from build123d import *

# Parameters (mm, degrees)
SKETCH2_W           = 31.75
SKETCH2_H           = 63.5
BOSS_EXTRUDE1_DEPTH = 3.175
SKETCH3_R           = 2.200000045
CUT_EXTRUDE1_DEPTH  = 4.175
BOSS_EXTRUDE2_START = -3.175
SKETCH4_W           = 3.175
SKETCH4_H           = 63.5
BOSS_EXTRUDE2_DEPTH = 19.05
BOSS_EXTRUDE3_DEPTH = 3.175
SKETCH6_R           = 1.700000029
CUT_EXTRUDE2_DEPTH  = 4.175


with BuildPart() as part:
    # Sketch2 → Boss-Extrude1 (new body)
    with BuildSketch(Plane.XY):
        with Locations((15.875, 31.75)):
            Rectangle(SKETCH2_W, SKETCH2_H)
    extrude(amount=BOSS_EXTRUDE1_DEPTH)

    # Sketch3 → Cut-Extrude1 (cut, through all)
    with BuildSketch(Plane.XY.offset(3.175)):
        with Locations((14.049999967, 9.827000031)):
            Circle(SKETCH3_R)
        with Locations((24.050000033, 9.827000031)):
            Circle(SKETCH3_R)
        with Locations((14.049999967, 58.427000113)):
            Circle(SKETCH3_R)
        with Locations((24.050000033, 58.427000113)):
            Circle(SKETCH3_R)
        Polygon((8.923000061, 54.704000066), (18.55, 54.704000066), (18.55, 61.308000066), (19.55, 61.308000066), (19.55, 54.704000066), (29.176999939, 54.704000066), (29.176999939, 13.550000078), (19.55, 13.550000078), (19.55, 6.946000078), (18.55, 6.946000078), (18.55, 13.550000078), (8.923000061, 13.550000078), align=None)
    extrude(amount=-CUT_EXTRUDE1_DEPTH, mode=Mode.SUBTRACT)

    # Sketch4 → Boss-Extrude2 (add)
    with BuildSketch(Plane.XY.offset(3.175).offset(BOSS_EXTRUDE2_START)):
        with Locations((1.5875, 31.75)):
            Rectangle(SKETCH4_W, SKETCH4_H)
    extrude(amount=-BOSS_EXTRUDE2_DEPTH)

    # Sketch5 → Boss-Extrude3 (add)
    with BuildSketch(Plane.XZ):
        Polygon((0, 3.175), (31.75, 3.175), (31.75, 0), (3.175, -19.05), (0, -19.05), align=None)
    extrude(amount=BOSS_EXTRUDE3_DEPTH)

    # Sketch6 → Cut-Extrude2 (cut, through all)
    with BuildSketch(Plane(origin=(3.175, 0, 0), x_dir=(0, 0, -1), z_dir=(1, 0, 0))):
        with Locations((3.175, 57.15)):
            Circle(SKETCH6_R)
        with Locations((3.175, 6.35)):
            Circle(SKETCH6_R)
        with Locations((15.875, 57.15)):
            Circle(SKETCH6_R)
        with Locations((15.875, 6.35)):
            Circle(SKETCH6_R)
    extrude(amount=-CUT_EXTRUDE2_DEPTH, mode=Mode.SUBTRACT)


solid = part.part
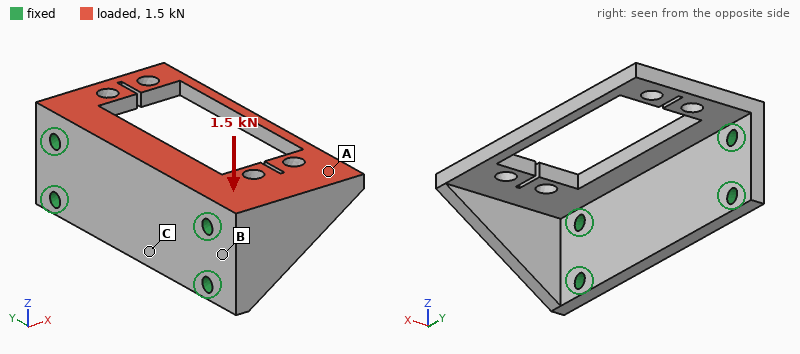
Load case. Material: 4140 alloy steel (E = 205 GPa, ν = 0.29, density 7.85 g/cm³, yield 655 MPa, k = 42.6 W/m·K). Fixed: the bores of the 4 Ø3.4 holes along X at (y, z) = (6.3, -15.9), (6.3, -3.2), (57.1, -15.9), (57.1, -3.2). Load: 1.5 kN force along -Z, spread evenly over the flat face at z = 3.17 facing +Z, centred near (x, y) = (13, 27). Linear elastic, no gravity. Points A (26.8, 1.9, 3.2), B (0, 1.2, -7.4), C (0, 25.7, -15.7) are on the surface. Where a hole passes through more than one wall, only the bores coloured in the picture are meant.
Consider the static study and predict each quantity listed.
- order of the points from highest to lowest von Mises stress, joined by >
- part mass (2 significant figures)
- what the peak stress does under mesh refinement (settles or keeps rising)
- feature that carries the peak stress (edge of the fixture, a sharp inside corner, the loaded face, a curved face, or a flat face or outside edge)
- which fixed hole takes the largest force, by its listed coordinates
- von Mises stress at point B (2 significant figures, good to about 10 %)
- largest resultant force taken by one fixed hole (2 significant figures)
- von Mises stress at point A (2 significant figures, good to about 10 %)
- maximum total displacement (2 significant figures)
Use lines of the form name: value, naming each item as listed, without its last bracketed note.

order of the points from highest to lowest von Mises stress, joined by >: A > B > C
part mass: 68 g
what the peak stress does under mesh refinement: keeps rising
feature that carries the peak stress: a sharp inside corner
which fixed hole takes the largest force, by its listed coordinates: (6.3, -3.2)
von Mises stress at point B: 59 MPa
largest resultant force taken by one fixed hole: 920 N
von Mises stress at point A: 89 MPa
maximum total displacement: 0.37 mm
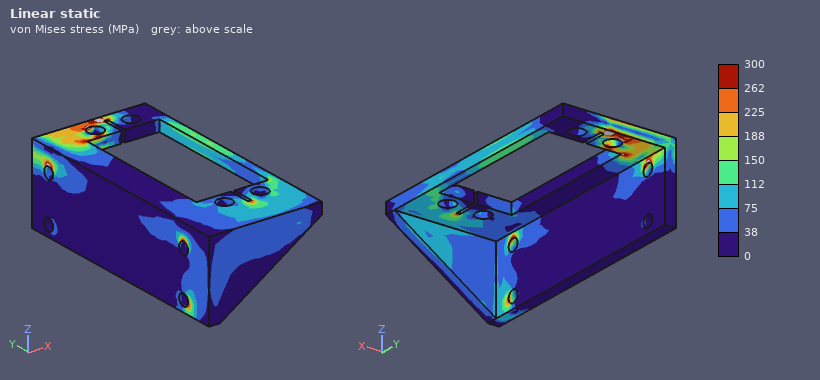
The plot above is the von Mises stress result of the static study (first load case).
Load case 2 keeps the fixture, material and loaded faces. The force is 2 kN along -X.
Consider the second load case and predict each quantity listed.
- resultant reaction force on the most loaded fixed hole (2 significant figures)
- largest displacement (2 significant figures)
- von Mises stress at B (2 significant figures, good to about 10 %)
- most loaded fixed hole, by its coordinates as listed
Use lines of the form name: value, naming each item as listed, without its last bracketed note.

resultant reaction force on the most loaded fixed hole: 1.5 kN
largest displacement: 0.10 mm
von Mises stress at B: 32 MPa
most loaded fixed hole, by its coordinates as listed: (6.3, -3.2)
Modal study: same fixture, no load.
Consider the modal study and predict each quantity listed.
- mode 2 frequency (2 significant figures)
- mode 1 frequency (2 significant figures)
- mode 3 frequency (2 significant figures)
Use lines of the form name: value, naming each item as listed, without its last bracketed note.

mode 2 frequency: 4300 Hz
mode 1 frequency: 2300 Hz
mode 3 frequency: 5100 Hz
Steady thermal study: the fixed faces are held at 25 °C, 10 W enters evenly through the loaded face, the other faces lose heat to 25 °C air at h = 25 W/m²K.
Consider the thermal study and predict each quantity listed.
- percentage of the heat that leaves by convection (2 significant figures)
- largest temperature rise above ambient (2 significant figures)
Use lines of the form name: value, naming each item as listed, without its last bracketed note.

percentage of the heat that leaves by convection: 17 %
largest temperature rise above ambient: 43 K
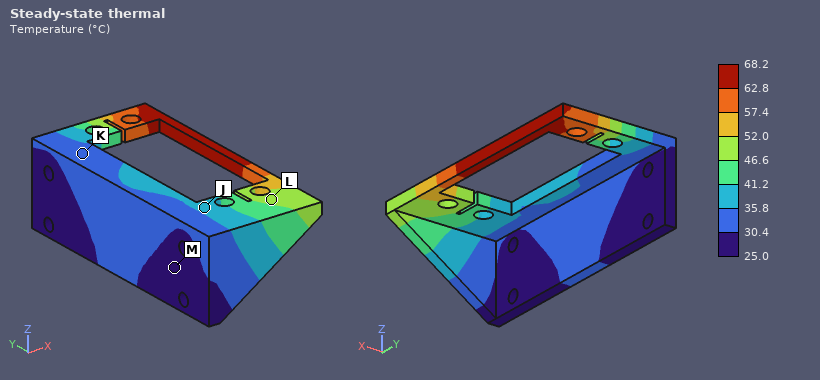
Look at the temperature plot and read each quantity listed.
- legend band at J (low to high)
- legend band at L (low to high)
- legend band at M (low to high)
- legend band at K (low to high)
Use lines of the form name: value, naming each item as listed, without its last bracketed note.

legend band at J: 35.8 to 41.2 °C
legend band at L: 46.6 to 52.0 °C
legend band at M: 25.0 to 30.4 °C
legend band at K: 30.4 to 35.8 °C
